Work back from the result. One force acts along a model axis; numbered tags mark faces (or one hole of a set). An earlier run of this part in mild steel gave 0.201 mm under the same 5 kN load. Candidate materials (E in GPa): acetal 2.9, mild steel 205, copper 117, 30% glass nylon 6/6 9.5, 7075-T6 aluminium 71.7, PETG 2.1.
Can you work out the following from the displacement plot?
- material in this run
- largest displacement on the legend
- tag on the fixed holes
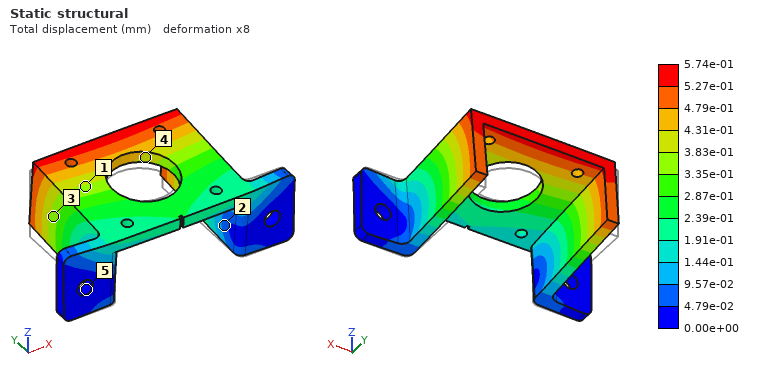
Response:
7075-T6 aluminium
5.74e-01 mm
5
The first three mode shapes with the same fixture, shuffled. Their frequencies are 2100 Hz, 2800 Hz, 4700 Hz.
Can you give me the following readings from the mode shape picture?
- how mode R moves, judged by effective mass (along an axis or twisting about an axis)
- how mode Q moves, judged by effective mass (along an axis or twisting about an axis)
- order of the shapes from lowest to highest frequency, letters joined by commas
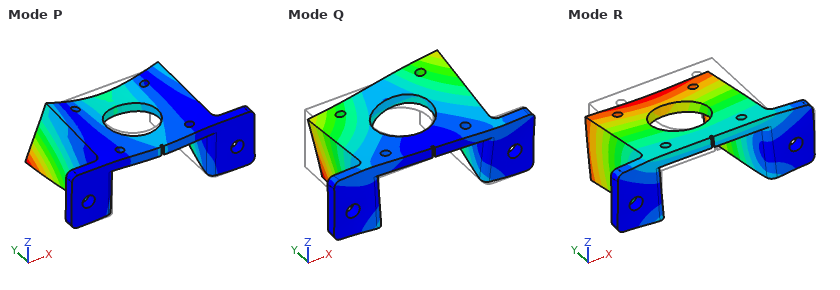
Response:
along Z
along X
R, Q, P
